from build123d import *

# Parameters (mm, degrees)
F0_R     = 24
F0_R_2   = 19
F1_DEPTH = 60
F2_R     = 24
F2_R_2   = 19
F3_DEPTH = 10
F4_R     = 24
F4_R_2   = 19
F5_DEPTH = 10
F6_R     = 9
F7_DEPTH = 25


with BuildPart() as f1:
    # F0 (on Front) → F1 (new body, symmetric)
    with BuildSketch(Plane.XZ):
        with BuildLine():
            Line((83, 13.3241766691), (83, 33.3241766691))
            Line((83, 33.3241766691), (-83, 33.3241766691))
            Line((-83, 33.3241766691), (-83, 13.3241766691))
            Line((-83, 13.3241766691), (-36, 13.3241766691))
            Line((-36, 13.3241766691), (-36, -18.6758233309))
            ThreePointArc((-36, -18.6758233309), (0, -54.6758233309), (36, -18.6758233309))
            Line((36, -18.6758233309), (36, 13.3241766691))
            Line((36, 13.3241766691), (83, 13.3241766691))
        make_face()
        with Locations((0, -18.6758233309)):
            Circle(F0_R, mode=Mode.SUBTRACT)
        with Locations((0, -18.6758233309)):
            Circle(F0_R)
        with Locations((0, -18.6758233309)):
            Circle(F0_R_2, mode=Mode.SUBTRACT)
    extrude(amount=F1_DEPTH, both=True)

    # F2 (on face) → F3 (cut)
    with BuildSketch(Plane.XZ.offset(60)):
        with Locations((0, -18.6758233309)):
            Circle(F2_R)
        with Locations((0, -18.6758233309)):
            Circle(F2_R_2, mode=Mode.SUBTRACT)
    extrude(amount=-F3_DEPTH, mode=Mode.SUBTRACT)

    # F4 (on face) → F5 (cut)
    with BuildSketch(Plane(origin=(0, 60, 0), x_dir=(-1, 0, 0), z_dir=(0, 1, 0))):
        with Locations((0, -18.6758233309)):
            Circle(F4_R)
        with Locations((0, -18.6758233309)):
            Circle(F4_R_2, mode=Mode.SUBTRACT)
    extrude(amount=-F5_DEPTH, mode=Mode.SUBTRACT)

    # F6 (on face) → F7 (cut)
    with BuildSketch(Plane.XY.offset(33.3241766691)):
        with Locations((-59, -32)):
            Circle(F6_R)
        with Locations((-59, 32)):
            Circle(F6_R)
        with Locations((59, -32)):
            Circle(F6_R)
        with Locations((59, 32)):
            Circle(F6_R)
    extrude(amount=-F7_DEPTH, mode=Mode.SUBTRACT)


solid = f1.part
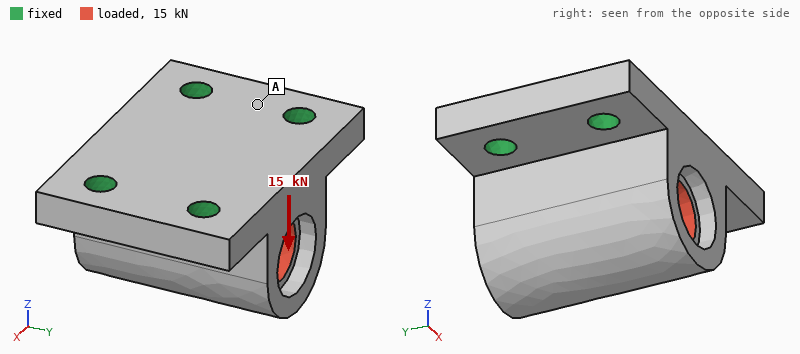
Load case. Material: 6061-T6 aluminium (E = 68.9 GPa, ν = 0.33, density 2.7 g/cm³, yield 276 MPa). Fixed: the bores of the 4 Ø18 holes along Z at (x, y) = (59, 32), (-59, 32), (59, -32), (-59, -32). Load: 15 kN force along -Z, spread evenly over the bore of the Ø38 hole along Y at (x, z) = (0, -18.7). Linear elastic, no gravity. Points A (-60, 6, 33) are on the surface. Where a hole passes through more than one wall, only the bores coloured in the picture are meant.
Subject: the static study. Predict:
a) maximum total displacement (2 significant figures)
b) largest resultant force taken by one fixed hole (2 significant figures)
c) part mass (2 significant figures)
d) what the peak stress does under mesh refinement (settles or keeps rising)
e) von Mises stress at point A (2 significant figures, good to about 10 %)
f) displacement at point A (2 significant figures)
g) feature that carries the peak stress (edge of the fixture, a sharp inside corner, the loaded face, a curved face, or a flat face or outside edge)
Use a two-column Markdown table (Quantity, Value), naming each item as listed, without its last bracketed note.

| Quantity | Value |
|---|---|
| maximum total displacement | 9.7 µm |
| largest resultant force taken by one fixed hole | 4.0 kN |
| part mass | 2.0 kg |
| what the peak stress does under mesh refinement | keeps rising |
| von Mises stress at point A | 3.4 MPa |
| displacement at point A | 1.9 µm |
| feature that carries the peak stress | edge of the fixture |
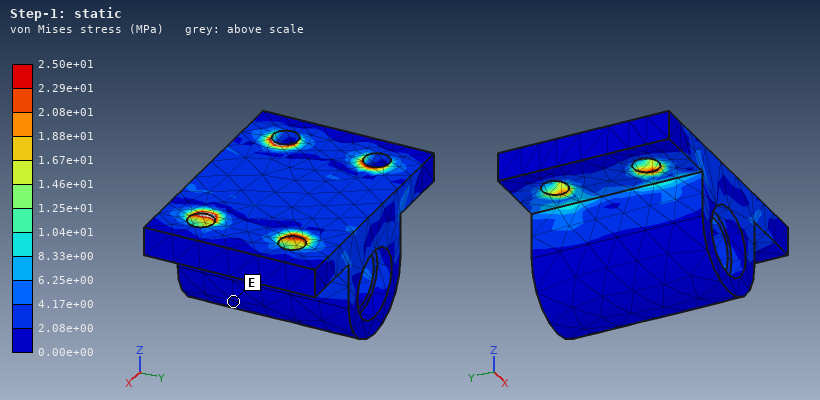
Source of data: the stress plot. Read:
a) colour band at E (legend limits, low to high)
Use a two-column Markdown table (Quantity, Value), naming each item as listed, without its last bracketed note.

| Quantity | Value |
|---|---|
| colour band at E | 0.00e+00 to 2.08e+00 MPa |
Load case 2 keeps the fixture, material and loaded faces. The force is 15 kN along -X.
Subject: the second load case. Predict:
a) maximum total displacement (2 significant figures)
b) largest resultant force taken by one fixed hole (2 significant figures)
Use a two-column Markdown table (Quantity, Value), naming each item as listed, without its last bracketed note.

| Quantity | Value |
|---|---|
| maximum total displacement | 22 µm |
| largest resultant force taken by one fixed hole | 5.1 kN |
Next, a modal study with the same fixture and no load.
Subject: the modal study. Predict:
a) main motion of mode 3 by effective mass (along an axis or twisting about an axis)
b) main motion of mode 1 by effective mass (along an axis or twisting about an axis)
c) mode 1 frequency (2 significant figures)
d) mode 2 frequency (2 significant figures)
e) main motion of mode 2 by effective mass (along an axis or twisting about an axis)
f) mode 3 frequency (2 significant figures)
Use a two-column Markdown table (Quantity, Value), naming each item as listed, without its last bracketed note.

| Quantity | Value |
|---|---|
| main motion of mode 3 by effective mass | along Z |
| main motion of mode 1 by effective mass | along Y |
| mode 1 frequency | 3800 Hz |
| mode 2 frequency | 4800 Hz |
| main motion of mode 2 by effective mass | along X |
| mode 3 frequency | 5600 Hz |
